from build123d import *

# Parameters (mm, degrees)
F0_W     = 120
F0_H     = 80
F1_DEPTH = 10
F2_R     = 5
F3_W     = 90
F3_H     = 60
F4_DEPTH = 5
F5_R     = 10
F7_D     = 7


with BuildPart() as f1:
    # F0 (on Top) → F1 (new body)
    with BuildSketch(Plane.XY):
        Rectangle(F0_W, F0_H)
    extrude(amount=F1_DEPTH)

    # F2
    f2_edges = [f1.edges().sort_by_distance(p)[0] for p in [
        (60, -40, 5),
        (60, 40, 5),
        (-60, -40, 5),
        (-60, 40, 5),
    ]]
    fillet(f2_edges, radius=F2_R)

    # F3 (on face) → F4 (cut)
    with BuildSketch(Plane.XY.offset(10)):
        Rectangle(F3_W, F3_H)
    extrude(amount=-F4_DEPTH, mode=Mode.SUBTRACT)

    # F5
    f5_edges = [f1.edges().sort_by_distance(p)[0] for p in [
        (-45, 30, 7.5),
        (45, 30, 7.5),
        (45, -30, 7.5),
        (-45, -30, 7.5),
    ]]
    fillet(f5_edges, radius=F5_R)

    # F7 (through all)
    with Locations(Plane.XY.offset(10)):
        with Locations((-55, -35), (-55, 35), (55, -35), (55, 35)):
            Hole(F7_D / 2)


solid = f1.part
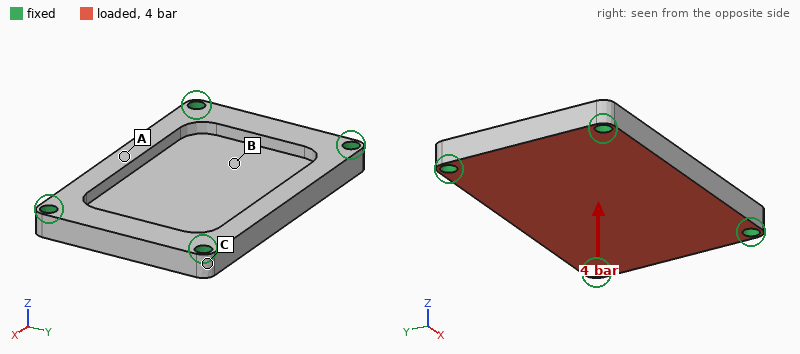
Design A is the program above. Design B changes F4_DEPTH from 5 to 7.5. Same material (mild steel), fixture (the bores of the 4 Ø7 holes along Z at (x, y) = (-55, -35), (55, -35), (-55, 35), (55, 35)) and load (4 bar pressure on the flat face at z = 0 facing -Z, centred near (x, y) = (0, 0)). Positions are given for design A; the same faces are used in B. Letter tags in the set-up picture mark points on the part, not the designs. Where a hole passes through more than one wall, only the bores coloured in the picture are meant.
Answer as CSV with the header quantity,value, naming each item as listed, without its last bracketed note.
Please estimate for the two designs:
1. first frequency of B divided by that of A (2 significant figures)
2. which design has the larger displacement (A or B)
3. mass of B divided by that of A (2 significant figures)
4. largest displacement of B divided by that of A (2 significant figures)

quantity,value
first frequency of B divided by that of A,0.94
which design has the larger displacement,B
mass of B divided by that of A,0.80
largest displacement of B divided by that of A,2.6
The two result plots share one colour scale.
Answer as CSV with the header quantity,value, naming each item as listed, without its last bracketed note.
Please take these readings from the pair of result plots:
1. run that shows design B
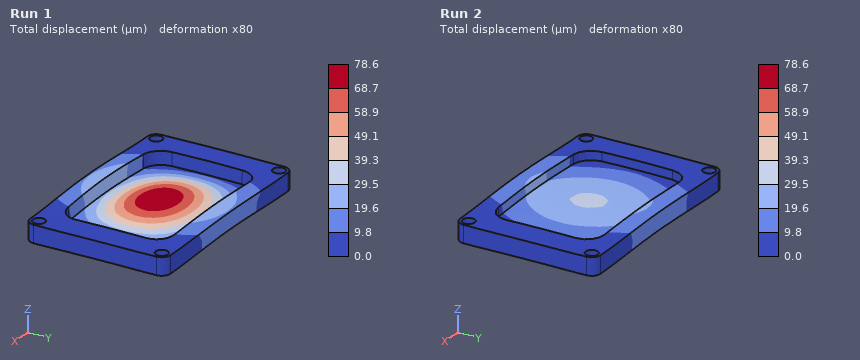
quantity,value
run that shows design B,Run 1
